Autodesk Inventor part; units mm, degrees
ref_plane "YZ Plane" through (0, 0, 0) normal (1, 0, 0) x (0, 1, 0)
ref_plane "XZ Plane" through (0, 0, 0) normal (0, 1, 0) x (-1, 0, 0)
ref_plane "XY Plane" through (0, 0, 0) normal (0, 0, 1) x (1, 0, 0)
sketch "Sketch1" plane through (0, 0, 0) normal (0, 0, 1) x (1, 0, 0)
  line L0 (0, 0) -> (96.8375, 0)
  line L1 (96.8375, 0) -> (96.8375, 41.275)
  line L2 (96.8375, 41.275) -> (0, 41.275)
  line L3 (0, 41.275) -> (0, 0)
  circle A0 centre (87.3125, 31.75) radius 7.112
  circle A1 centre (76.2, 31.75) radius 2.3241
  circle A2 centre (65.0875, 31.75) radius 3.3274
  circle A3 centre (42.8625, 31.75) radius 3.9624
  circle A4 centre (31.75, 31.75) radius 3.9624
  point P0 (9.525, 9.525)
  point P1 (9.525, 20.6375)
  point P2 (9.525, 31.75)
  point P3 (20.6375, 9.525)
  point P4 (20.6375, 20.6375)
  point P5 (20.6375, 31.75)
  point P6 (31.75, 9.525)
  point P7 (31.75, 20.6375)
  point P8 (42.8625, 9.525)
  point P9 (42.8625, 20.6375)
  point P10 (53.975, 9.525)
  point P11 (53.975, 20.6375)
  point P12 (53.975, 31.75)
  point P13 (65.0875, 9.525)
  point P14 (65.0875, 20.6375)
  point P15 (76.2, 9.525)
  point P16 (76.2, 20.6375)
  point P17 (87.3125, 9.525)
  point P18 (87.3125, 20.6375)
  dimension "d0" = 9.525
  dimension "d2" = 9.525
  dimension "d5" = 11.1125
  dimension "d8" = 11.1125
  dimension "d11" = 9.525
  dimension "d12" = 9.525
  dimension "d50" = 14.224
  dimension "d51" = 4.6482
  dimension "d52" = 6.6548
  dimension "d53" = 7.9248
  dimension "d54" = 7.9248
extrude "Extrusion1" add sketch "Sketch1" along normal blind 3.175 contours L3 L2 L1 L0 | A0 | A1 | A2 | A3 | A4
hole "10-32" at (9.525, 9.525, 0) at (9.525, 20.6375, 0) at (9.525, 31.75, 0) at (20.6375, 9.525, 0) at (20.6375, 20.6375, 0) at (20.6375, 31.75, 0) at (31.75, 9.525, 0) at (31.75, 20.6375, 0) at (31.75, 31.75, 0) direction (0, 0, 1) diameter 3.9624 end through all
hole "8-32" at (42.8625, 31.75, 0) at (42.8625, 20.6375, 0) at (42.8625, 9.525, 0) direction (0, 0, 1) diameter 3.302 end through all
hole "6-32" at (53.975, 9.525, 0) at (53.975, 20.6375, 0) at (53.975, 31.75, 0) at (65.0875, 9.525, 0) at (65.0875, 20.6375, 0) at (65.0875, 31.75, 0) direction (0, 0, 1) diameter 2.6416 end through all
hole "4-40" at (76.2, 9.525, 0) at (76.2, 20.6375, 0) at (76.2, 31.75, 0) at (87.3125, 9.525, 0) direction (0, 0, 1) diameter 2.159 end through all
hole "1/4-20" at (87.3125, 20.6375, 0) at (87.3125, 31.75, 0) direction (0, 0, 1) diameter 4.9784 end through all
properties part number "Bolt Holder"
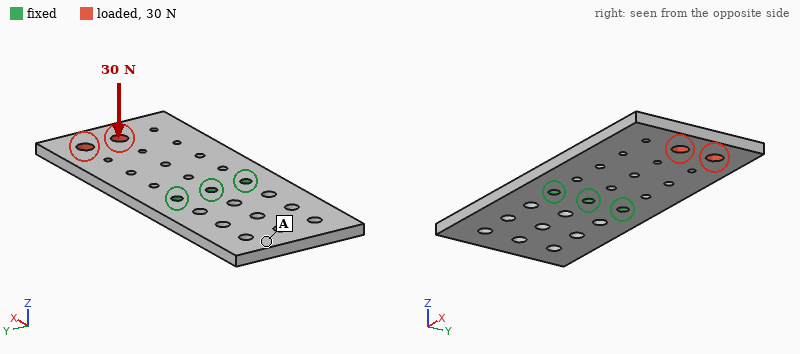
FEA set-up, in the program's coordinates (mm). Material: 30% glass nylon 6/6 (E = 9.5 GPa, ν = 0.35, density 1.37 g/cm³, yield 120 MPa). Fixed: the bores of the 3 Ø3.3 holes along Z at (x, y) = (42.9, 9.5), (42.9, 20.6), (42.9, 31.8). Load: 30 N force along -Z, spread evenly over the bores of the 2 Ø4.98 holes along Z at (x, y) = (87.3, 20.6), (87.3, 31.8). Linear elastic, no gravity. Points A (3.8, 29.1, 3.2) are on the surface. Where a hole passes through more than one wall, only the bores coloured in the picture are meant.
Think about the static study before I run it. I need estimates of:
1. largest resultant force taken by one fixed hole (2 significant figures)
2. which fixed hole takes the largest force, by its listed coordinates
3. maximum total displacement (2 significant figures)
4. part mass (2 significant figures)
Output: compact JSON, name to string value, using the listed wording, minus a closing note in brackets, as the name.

{"largest resultant force taken by one fixed hole": "20 N", "which fixed hole takes the largest force, by its listed coordinates": "(42.9, 20.6)", "maximum total displacement": "1.2 mm", "part mass": "16 g"}
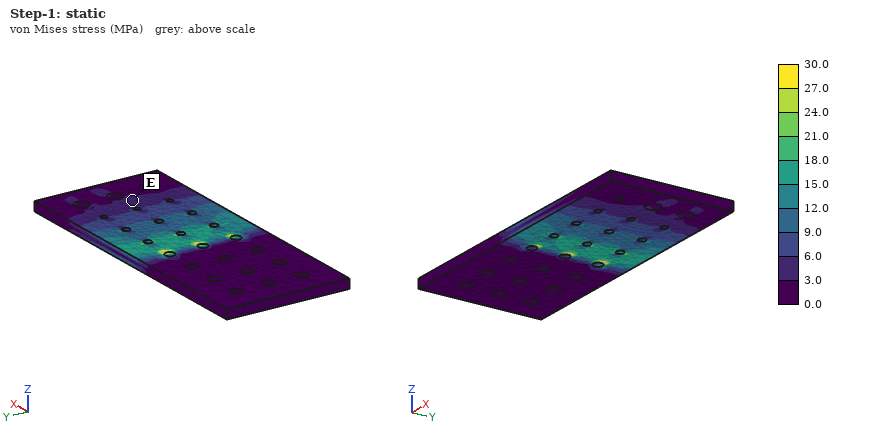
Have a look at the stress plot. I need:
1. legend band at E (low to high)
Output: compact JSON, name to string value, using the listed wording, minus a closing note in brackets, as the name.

{"legend band at E": "3.0 to 6.0 MPa"}
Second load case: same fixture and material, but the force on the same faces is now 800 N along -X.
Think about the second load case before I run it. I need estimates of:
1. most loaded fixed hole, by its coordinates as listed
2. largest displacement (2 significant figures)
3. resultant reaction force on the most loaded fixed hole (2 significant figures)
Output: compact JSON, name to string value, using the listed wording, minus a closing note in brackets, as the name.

{"most loaded fixed hole, by its coordinates as listed": "(42.9, 31.8)", "largest displacement": "67 µm", "resultant reaction force on the most loaded fixed hole": "480 N"}
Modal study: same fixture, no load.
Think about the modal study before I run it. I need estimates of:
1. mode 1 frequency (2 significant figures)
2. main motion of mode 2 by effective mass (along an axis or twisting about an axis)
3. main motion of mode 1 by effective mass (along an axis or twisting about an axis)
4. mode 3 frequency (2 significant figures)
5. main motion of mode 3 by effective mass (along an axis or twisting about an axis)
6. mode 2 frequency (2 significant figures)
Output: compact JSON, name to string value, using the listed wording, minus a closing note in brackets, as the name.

{"mode 1 frequency": "480 Hz", "main motion of mode 2 by effective mass": "along Z", "main motion of mode 1 by effective mass": "along Z", "mode 3 frequency": "1300 Hz", "main motion of mode 3 by effective mass": "twisting about X", "mode 2 frequency": "750 Hz"}
